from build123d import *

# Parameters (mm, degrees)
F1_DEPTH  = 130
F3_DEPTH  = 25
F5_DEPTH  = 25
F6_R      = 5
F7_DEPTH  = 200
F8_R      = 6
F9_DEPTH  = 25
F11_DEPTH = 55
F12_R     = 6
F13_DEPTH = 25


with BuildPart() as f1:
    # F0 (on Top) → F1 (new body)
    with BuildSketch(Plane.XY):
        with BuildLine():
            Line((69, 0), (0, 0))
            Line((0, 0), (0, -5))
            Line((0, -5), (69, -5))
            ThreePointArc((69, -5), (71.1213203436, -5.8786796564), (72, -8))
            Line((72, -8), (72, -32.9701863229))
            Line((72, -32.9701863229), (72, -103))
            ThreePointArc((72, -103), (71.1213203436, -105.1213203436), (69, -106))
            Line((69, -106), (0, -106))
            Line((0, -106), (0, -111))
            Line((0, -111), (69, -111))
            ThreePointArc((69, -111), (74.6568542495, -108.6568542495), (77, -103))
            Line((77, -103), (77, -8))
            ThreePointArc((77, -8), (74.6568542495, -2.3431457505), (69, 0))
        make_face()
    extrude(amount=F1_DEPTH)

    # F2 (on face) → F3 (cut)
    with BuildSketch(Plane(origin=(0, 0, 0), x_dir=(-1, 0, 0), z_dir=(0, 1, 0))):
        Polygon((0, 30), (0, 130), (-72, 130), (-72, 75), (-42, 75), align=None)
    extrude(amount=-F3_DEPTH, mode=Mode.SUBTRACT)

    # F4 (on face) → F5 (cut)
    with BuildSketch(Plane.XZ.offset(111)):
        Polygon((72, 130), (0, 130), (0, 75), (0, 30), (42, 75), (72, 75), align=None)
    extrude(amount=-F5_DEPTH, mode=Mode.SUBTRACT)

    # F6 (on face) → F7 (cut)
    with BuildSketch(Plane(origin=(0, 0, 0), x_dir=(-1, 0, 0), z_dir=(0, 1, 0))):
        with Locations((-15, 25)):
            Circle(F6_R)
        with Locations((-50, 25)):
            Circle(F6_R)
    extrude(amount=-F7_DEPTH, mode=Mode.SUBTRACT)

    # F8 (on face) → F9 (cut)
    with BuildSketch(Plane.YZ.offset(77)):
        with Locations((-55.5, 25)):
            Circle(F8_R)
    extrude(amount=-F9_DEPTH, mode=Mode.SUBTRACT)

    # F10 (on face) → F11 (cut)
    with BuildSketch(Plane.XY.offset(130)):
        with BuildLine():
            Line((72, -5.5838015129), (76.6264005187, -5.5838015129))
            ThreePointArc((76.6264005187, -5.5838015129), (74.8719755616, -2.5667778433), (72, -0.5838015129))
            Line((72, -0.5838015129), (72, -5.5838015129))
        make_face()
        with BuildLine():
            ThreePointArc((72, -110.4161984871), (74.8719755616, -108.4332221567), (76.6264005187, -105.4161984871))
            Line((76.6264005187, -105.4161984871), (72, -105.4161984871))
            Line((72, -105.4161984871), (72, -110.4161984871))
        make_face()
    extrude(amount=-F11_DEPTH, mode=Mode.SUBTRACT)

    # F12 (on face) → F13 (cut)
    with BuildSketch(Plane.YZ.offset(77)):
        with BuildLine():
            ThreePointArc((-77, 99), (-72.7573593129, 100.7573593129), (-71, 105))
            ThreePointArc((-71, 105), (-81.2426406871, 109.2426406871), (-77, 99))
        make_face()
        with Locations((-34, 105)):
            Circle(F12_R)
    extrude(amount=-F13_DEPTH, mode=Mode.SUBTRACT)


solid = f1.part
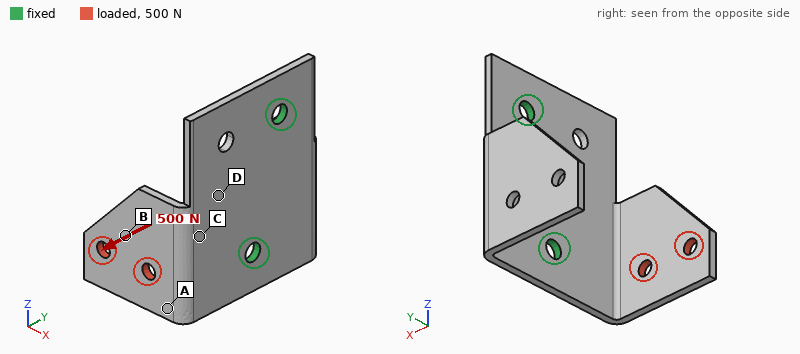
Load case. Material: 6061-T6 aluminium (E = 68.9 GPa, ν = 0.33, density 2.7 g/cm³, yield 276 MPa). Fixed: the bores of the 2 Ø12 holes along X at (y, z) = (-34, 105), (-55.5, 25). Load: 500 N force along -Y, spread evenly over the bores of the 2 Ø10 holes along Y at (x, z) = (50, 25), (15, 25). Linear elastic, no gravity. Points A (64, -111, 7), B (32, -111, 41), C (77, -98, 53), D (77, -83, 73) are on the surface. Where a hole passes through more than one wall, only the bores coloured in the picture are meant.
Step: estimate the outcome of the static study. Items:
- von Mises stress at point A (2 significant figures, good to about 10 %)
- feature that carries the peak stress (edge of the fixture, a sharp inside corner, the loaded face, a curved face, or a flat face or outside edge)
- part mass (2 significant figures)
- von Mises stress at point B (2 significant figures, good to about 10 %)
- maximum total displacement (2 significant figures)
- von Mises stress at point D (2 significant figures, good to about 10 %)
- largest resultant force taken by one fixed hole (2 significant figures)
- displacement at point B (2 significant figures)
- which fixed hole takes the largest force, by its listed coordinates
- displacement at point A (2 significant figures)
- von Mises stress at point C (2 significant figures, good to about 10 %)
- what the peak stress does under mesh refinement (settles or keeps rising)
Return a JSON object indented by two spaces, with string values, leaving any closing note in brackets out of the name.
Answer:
{
  "von Mises stress at point A": "47 MPa",
  "feature that carries the peak stress": "edge of the fixture",
  "part mass": "290 g",
  "von Mises stress at point B": "24 MPa",
  "maximum total displacement": "1.9 mm",
  "von Mises stress at point D": "34 MPa",
  "largest resultant force taken by one fixed hole": "480 N",
  "displacement at point B": "0.99 mm",
  "which fixed hole takes the largest force, by its listed coordinates": "(-55.5, 25)",
  "displacement at point A": "0.53 mm",
  "von Mises stress at point C": "54 MPa",
  "what the peak stress does under mesh refinement": "keeps rising"
}
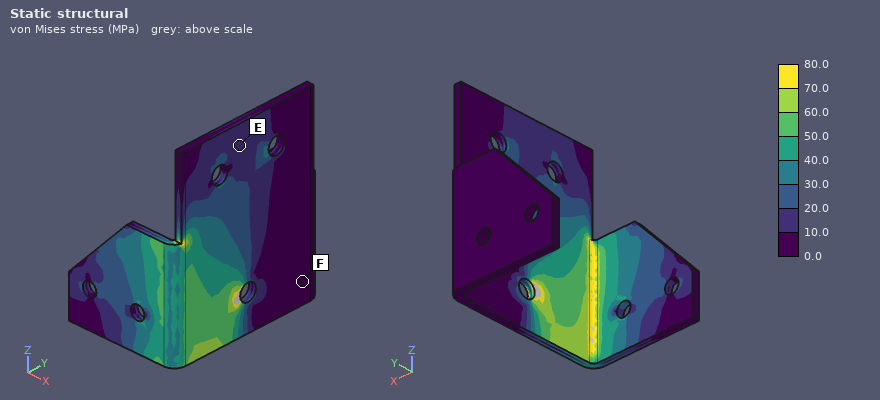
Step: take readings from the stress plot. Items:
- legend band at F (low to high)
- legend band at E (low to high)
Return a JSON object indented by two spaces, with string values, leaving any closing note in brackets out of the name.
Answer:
{
  "legend band at F": "0.0 to 10.0 MPa",
  "legend band at E": "10.0 to 20.0 MPa"
}
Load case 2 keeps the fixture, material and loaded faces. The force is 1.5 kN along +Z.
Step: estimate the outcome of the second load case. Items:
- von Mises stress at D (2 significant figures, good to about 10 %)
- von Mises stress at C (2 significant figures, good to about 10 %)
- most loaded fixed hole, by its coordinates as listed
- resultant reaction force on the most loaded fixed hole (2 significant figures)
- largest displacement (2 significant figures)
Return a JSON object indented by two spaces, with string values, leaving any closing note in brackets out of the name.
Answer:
{
  "von Mises stress at D": "76 MPa",
  "von Mises stress at C": "85 MPa",
  "most loaded fixed hole, by its coordinates as listed": "(-55.5, 25)",
  "resultant reaction force on the most loaded fixed hole": "1.6 kN",
  "largest displacement": "1.7 mm"
}
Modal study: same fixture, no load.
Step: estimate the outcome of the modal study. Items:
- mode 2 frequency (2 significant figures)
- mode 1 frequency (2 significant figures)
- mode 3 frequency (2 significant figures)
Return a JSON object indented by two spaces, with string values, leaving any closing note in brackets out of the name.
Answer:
{
  "mode 2 frequency": "480 Hz",
  "mode 1 frequency": "440 Hz",
  "mode 3 frequency": "740 Hz"
}
